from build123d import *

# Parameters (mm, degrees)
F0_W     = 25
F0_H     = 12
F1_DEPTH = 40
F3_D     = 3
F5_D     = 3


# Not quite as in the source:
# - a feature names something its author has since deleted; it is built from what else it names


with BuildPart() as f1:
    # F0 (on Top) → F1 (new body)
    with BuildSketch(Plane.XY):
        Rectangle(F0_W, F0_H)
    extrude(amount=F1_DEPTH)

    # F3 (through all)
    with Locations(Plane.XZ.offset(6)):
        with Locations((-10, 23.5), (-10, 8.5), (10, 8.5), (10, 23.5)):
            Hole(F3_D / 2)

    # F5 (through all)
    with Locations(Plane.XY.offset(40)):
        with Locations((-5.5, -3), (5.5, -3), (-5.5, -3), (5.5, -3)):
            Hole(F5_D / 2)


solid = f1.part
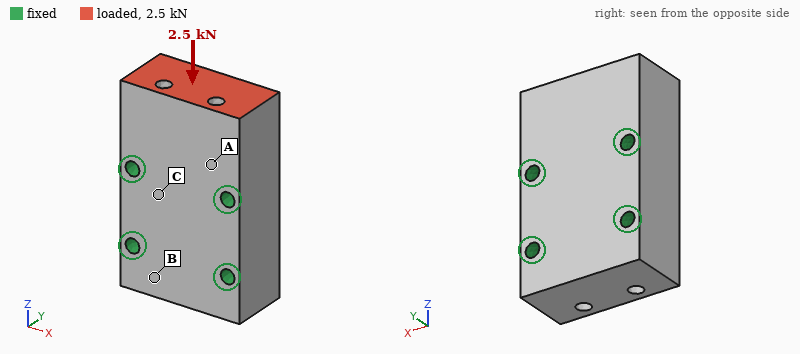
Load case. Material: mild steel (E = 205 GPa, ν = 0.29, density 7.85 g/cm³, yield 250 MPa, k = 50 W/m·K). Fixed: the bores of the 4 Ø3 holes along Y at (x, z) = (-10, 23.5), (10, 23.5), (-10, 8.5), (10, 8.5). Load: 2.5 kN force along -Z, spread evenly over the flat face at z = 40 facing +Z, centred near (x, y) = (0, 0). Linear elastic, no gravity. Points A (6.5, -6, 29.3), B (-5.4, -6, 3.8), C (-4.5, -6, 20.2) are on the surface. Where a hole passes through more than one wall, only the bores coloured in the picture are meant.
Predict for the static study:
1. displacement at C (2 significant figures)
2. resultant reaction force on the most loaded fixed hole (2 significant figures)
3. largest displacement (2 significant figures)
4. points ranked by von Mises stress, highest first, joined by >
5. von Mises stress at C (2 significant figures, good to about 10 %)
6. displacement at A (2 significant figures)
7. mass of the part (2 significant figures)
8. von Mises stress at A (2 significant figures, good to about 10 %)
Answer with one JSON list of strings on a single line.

["0.19 µm", "1.1 kN", "0.84 µm", "A > C > B", "5.0 MPa", "0.35 µm", "87 g", "9.2 MPa"]
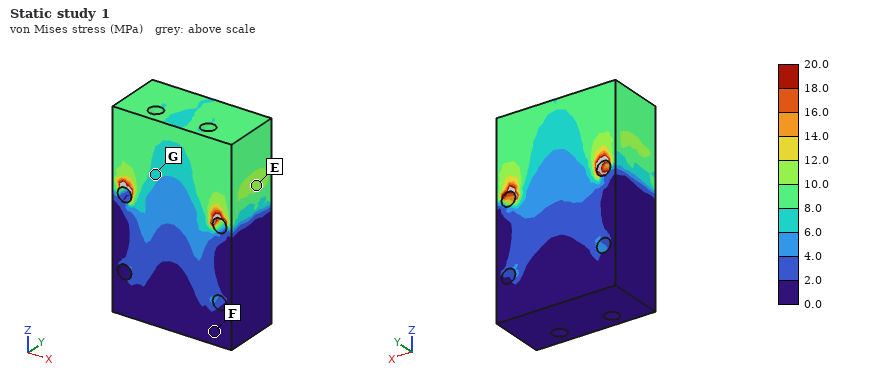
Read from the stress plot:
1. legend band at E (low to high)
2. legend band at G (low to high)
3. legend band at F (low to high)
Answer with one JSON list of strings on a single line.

["10.0 to 12.0 MPa", "6.0 to 8.0 MPa", "0.0 to 2.0 MPa"]
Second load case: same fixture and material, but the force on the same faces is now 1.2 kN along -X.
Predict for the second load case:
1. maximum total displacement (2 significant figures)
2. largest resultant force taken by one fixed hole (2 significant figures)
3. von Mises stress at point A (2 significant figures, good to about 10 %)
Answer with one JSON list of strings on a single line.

["2.0 µm", "1.1 kN", "12 MPa"]
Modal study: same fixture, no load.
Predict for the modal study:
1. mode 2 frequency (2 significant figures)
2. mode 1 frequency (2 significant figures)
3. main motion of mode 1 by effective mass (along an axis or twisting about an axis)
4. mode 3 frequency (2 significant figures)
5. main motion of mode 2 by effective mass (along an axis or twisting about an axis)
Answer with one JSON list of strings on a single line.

["37 kHz", "24 kHz", "along Y", "40 kHz", "along X"]
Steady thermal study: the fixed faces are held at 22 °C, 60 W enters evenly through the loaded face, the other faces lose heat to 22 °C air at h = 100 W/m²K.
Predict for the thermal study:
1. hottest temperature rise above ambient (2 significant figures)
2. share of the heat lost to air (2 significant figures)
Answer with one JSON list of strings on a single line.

["70 K", "9.9 %"]
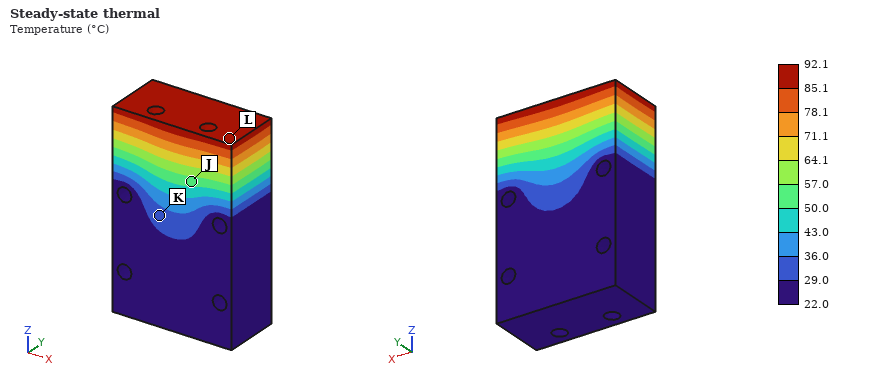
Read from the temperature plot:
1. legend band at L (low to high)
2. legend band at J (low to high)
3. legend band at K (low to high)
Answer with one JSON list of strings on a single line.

["85.1 to 92.1 °C", "50.0 to 57.0 °C", "29.0 to 36.0 °C"]
